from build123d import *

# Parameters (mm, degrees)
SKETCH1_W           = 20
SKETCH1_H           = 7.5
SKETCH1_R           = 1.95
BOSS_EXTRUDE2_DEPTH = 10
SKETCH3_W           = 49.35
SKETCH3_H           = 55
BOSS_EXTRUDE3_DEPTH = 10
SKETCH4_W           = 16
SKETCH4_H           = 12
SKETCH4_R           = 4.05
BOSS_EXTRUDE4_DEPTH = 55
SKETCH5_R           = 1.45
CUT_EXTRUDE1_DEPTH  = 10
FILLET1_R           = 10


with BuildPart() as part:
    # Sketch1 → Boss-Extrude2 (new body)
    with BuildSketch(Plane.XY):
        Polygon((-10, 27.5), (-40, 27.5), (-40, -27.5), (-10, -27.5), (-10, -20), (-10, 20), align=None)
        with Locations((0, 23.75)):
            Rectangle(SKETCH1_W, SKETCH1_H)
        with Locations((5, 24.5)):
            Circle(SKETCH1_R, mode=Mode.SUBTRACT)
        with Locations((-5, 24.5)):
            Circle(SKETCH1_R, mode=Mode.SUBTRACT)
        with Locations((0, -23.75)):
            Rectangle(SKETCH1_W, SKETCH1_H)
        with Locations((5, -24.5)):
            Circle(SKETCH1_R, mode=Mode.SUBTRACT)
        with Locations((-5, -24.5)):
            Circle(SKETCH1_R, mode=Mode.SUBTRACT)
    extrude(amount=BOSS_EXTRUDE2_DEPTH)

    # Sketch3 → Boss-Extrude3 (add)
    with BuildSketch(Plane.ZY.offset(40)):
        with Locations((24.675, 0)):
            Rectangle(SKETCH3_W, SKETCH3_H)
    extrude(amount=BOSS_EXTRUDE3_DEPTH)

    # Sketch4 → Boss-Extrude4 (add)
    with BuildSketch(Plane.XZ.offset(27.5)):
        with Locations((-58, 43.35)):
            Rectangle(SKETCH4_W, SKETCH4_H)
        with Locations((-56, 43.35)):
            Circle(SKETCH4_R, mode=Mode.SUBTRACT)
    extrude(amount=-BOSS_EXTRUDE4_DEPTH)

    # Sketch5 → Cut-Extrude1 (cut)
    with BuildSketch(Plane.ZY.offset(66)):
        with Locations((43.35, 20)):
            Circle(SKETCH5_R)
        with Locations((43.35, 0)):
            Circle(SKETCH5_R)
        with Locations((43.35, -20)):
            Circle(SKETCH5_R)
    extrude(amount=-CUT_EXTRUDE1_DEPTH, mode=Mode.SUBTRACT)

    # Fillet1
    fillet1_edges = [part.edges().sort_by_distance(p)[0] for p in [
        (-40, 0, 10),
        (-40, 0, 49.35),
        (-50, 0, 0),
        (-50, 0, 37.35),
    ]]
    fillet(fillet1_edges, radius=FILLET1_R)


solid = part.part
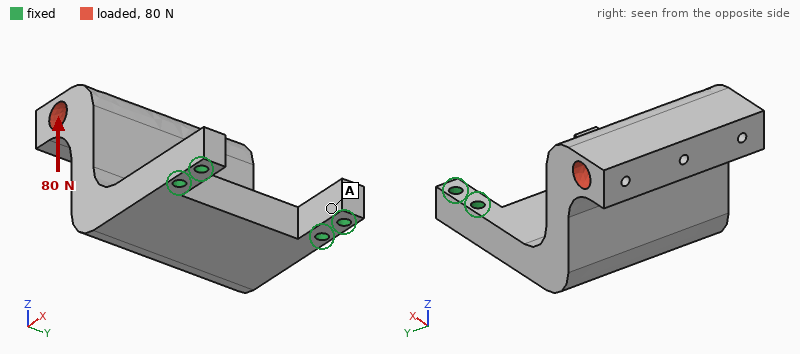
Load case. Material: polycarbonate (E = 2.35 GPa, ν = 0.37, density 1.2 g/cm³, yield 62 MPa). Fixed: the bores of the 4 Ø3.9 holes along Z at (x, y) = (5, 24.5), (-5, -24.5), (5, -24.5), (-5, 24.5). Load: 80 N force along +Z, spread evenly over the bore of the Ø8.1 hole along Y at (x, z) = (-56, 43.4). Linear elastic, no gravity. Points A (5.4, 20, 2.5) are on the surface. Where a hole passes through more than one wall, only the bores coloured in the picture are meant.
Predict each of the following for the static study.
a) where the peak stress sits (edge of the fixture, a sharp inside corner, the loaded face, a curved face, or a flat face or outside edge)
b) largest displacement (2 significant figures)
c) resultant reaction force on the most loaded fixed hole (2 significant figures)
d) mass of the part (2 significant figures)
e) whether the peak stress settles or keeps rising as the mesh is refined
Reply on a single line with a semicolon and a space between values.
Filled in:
edge of the fixture; 1.3 mm; 48 N; 65 g; keeps rising
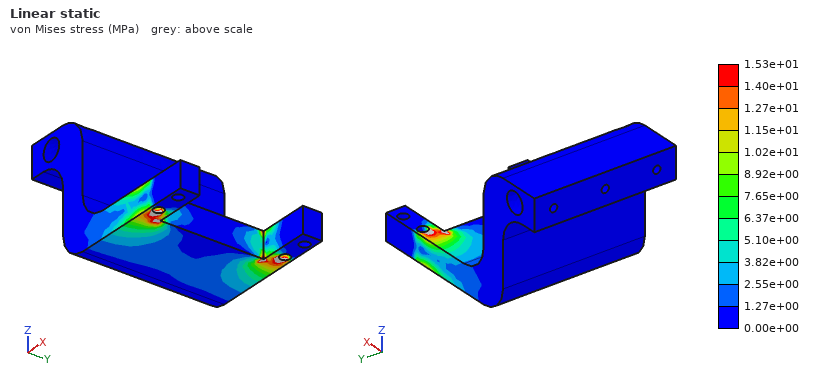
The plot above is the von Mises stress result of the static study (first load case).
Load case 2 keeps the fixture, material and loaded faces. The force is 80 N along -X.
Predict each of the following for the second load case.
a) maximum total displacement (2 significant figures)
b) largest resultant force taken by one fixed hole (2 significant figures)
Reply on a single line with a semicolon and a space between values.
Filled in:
1.3 mm; 42 N
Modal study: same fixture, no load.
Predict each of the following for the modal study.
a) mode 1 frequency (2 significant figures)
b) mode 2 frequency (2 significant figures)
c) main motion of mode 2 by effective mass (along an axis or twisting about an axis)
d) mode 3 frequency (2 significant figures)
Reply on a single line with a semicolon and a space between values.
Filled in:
230 Hz; 630 Hz; along Y; 1100 Hz
